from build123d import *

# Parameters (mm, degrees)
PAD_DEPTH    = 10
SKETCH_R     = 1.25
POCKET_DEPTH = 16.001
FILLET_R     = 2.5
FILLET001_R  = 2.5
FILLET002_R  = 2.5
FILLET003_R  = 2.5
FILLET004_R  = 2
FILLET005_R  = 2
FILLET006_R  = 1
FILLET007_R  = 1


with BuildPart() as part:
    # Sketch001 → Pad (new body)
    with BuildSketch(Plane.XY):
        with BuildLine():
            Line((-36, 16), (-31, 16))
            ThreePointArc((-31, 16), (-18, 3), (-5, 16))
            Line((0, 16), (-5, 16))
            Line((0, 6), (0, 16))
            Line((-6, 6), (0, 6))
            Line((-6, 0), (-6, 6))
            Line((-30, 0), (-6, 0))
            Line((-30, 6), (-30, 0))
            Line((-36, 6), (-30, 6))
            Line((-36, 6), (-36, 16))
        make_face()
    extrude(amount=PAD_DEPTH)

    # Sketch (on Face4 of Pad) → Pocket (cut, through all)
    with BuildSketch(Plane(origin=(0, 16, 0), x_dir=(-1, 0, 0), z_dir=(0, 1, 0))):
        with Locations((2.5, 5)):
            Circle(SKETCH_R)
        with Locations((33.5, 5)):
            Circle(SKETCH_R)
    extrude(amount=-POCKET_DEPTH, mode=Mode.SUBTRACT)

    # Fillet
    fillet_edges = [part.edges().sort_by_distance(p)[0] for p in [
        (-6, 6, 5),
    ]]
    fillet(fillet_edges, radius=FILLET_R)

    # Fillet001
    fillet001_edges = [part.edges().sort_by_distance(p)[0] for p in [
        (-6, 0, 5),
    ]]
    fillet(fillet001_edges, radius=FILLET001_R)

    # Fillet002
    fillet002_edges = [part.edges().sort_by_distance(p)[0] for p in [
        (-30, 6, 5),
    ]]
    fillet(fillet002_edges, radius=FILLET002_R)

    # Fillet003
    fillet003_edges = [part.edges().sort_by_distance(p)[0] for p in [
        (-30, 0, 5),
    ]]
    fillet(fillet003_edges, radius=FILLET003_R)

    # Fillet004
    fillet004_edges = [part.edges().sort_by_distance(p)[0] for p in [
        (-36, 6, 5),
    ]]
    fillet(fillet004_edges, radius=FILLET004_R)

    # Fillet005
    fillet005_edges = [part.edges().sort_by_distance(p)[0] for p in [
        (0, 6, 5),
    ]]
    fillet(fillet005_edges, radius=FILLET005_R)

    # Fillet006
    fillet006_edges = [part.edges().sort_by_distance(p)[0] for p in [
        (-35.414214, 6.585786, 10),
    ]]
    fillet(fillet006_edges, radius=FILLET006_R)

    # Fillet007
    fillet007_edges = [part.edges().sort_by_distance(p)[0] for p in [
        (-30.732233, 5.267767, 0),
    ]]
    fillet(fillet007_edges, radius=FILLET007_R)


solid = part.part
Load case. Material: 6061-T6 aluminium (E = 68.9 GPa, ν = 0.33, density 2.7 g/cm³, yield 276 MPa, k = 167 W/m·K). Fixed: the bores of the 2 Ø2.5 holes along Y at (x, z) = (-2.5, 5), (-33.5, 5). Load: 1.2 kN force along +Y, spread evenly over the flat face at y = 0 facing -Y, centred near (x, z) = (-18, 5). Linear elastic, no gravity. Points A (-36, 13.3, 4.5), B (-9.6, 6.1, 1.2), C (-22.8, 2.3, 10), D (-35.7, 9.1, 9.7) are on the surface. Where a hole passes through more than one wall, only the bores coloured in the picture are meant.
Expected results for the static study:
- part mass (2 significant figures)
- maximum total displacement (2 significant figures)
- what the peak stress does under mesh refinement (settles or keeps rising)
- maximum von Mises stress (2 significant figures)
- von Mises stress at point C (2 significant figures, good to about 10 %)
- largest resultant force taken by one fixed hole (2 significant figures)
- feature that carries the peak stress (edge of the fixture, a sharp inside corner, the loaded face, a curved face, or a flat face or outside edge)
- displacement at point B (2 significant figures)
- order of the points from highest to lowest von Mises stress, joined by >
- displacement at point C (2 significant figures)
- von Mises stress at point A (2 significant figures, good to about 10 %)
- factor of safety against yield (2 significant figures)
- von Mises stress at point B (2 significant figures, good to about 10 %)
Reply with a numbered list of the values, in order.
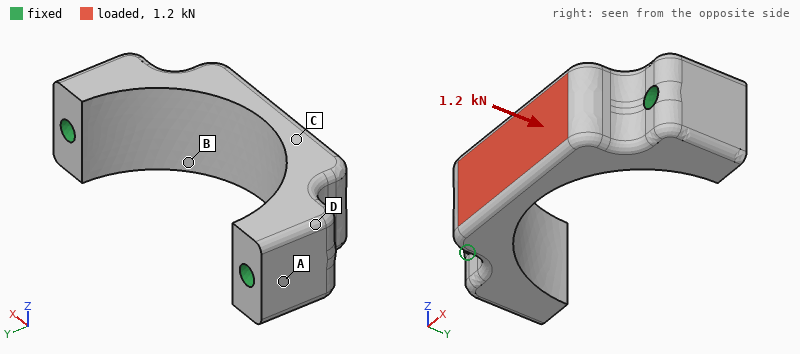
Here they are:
1. 6.1 g
2. 13 µm
3. settles
4. 55 MPa
5. 23 MPa
6. 880 N
7. the loaded face
8. 4.4 µm
9. B > C > A > D
10. 8.9 µm
11. 9.3 MPa
12. 5.1
13. 41 MPa
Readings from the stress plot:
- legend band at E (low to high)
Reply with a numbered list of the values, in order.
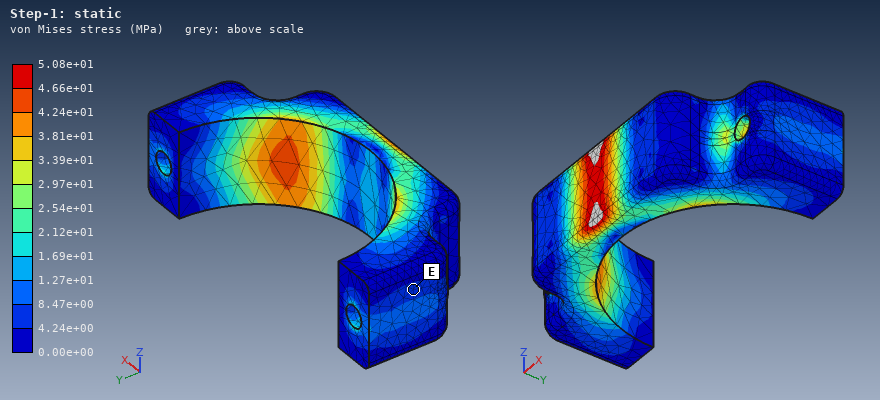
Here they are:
1. 4.24e+00 to 8.47e+00 MPa
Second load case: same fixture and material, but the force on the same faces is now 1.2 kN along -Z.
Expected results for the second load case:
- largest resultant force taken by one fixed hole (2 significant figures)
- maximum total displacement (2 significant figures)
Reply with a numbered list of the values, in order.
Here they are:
1. 600 N
2. 40 µm
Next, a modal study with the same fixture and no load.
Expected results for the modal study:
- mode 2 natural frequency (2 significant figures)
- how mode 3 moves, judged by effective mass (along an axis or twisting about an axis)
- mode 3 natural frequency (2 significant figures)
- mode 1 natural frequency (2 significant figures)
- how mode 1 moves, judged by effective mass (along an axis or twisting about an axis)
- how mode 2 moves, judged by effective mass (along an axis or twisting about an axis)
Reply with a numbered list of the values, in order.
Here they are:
1. 36 kHz
2. along Y
3. 39 kHz
4. 22 kHz
5. along Z
6. along X
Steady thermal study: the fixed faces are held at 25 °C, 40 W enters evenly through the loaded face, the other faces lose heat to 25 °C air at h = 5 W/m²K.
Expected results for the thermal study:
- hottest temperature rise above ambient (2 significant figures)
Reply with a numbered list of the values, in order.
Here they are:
1. 38 K
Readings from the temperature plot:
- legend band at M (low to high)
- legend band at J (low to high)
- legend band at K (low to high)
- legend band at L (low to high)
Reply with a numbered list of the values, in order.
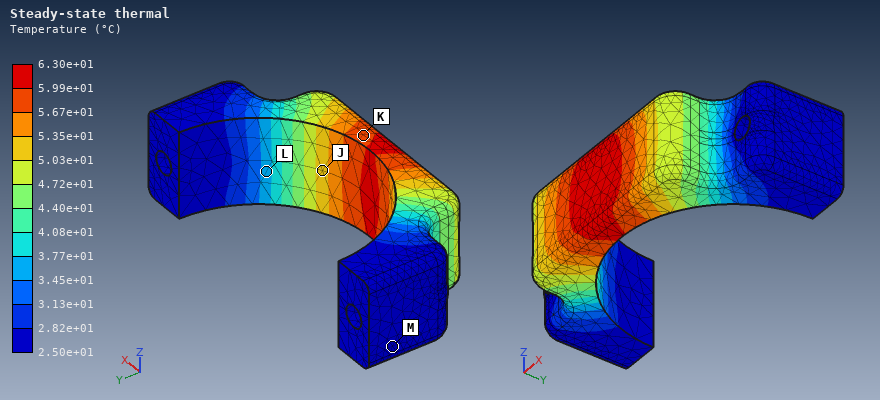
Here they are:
1. 2.50e+01 to 2.82e+01 °C
2. 5.03e+01 to 5.35e+01 °C
3. 5.67e+01 to 5.99e+01 °C
4. 3.45e+01 to 3.77e+01 °C
